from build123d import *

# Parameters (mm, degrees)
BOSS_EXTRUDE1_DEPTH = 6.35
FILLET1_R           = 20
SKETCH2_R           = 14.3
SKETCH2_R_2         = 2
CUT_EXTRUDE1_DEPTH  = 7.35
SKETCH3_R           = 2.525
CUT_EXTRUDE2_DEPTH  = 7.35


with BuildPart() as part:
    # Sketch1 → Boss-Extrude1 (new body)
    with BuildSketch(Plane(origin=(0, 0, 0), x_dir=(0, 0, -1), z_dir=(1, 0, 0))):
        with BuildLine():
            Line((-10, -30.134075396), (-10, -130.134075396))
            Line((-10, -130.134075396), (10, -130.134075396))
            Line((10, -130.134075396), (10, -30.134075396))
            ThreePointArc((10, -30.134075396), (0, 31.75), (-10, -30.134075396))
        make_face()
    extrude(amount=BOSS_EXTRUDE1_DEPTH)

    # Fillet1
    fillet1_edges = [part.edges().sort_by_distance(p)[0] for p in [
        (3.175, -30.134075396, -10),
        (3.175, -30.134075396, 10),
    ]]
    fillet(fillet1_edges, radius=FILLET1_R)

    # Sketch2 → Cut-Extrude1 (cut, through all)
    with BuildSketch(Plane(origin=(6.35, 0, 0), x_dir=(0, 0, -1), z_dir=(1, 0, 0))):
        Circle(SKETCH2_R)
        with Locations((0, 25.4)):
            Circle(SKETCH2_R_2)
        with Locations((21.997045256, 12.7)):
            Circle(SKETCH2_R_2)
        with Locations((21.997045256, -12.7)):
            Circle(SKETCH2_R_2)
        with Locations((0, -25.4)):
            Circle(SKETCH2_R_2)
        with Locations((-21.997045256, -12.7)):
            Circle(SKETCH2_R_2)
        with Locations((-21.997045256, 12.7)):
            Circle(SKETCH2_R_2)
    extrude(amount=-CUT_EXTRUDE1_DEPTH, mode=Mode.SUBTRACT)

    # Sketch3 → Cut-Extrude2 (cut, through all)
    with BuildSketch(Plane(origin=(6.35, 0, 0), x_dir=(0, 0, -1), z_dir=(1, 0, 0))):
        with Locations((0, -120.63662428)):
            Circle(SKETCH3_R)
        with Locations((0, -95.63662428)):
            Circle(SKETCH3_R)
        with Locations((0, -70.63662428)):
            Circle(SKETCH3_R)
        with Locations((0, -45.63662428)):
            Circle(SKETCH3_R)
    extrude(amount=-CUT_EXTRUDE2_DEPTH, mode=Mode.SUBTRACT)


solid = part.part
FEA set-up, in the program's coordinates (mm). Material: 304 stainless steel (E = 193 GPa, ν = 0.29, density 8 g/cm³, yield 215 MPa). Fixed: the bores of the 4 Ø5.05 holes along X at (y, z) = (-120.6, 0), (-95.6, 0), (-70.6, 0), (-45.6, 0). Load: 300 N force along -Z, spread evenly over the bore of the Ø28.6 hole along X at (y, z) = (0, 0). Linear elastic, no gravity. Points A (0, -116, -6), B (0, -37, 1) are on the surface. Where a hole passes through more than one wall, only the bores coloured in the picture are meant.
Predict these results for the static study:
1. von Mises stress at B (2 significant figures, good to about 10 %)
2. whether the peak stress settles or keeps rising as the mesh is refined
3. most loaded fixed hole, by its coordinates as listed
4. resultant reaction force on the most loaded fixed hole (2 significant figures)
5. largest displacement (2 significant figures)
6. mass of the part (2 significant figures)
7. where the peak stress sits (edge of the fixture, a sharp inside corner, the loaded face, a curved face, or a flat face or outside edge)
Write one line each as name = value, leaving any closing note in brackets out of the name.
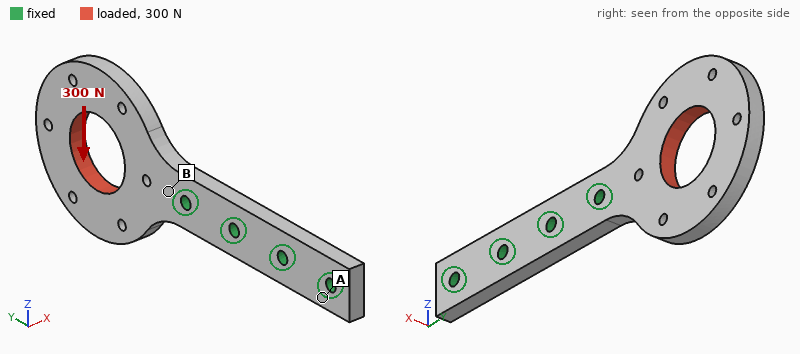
von Mises stress at B = 11 MPa
whether the peak stress settles or keeps rising as the mesh is refined = keeps rising
most loaded fixed hole, by its coordinates as listed = (-45.6, 0)
resultant reaction force on the most loaded fixed hole = 630 N
largest displacement = 29 µm
mass of the part = 220 g
where the peak stress sits = edge of the fixture
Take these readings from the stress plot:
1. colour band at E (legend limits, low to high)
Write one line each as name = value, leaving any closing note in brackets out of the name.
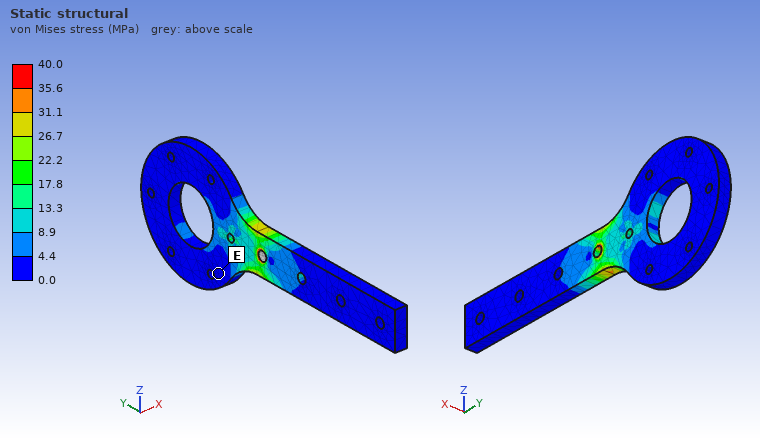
colour band at E = 0.0 to 4.4 MPa
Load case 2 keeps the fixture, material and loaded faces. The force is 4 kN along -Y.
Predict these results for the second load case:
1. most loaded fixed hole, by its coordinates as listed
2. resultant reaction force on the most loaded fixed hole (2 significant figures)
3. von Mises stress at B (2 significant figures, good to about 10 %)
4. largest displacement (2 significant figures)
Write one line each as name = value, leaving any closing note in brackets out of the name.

most loaded fixed hole, by its coordinates as listed = (-45.6, 0)
resultant reaction force on the most loaded fixed hole = 3.5 kN
von Mises stress at B = 30 MPa
largest displacement = 12 µm
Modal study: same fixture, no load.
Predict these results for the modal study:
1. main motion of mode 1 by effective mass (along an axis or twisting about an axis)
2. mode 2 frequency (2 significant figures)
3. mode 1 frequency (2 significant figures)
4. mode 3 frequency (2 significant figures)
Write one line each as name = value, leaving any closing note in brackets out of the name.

main motion of mode 1 by effective mass = along X
mode 2 frequency = 1600 Hz
mode 1 frequency = 670 Hz
mode 3 frequency = 1600 Hz
